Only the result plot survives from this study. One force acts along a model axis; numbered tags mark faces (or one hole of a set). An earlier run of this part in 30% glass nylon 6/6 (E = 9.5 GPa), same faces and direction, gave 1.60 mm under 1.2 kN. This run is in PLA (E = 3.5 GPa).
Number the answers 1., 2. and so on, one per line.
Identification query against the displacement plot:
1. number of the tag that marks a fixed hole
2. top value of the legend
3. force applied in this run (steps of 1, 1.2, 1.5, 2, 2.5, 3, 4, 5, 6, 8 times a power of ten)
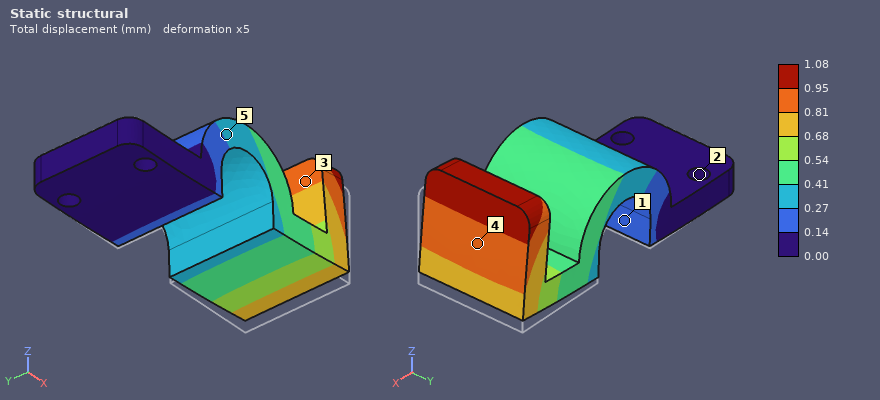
1. 2
2. 1.08 mm
3. 300 N
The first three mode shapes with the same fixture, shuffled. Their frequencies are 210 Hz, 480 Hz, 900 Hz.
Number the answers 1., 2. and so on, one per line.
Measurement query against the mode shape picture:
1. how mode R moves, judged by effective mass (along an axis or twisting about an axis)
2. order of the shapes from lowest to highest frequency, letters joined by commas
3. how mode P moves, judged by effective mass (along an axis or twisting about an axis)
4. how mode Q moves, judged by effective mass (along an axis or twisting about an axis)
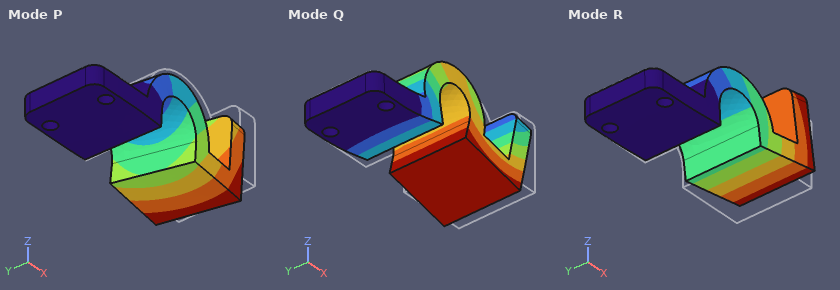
1. along Z
2. R, P, Q
3. along Y
4. along X
